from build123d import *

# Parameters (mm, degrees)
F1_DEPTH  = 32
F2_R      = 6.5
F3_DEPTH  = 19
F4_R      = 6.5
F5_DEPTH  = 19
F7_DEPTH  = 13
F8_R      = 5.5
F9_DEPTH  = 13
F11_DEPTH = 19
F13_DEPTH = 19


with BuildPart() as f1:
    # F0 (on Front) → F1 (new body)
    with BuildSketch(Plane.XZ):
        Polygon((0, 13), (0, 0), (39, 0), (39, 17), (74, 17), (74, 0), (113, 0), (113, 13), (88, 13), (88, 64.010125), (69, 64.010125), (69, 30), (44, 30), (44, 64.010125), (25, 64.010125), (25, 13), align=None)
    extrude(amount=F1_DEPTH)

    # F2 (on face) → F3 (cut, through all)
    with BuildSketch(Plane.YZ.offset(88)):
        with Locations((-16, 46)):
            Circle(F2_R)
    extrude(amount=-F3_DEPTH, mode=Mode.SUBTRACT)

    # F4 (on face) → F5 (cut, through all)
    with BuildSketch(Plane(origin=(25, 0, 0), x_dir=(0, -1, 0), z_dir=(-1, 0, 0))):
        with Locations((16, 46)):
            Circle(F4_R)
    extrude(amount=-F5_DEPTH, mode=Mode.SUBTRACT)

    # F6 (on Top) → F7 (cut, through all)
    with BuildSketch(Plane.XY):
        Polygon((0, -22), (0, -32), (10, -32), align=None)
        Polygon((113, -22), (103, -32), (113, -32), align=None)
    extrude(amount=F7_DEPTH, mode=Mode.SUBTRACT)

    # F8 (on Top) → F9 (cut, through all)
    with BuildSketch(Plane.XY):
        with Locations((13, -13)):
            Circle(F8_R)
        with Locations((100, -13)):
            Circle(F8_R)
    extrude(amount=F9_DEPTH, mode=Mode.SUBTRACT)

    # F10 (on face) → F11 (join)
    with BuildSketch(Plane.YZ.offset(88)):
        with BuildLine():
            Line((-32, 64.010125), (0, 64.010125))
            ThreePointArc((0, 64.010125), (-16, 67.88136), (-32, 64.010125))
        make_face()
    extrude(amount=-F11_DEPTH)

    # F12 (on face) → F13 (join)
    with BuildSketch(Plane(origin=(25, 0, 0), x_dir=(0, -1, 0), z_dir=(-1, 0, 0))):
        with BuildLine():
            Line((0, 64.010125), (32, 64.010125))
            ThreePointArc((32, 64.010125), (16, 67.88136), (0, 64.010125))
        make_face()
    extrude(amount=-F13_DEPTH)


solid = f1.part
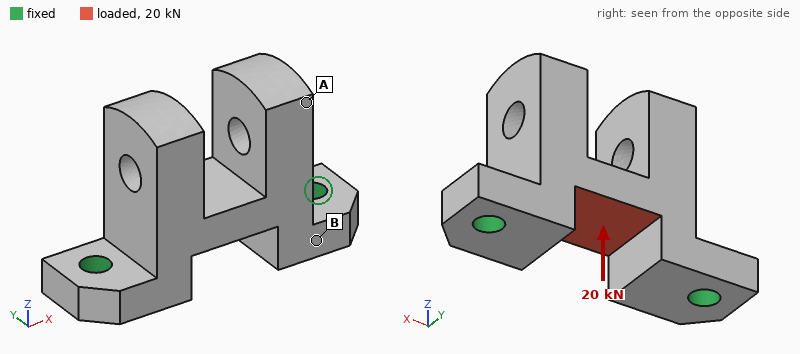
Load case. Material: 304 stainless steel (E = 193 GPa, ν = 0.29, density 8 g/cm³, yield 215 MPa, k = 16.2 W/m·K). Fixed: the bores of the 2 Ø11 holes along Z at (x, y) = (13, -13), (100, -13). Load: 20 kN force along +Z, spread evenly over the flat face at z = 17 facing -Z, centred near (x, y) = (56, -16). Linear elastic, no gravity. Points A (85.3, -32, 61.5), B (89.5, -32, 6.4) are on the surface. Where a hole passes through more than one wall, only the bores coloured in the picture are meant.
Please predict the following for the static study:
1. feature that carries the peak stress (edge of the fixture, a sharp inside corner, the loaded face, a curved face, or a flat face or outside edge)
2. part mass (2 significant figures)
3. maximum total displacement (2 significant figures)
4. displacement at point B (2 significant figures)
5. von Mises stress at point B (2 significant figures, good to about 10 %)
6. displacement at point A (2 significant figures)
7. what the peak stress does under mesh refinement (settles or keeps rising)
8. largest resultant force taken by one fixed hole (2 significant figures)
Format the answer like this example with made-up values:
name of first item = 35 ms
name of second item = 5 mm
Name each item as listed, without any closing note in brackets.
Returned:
feature that carries the peak stress = edge of the fixture
part mass = 780 g
maximum total displacement = 36 µm
displacement at point B = 10.0 µm
von Mises stress at point B = 32 MPa
displacement at point A = 29 µm
what the peak stress does under mesh refinement = keeps rising
largest resultant force taken by one fixed hole = 14 kN
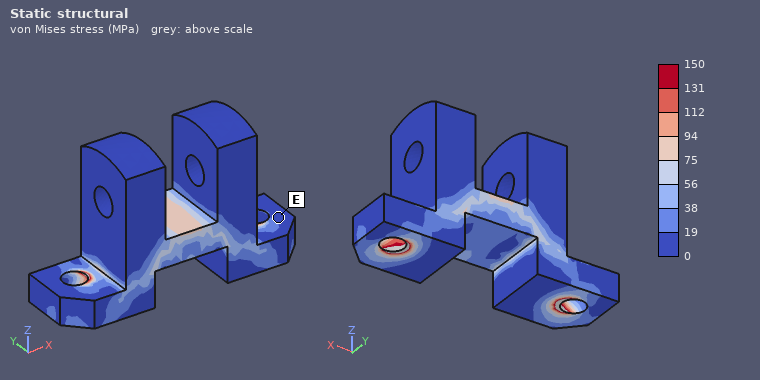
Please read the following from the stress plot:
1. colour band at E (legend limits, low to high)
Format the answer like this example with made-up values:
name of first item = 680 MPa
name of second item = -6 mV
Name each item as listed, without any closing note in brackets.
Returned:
colour band at E = 0 to 19 MPa
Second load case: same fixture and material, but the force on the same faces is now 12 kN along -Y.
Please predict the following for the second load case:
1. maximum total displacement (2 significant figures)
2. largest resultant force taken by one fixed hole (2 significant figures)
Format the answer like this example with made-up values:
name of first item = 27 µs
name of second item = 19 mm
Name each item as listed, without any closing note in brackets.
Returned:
maximum total displacement = 46 µm
largest resultant force taken by one fixed hole = 6.0 kN
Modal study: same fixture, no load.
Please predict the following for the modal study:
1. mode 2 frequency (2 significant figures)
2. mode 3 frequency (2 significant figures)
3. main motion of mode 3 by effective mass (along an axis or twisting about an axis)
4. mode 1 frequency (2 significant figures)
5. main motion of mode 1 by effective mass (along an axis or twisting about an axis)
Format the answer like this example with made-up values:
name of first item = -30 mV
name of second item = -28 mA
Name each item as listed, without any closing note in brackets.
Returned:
mode 2 frequency = 4000 Hz
mode 3 frequency = 4800 Hz
main motion of mode 3 by effective mass = along X
mode 1 frequency = 2500 Hz
main motion of mode 1 by effective mass = along Y
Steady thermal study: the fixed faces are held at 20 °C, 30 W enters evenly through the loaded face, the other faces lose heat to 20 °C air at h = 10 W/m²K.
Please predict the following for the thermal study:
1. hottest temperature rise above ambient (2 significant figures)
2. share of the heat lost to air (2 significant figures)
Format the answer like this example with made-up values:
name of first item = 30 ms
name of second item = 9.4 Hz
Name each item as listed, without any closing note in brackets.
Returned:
hottest temperature rise above ambient = 74 K
share of the heat lost to air = 23 %
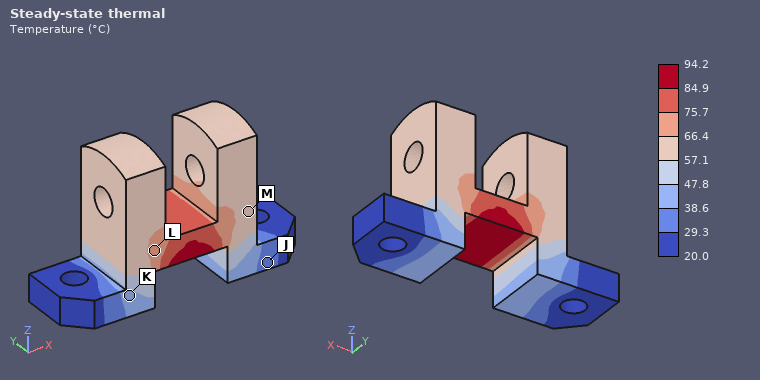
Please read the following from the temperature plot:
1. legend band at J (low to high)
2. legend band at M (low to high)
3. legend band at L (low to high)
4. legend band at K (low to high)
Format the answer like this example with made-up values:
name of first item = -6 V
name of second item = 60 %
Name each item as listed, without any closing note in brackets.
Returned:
legend band at J = 29.3 to 38.6 °C
legend band at M = 57.1 to 66.4 °C
legend band at L = 66.4 to 75.7 °C
legend band at K = 38.6 to 47.8 °C
